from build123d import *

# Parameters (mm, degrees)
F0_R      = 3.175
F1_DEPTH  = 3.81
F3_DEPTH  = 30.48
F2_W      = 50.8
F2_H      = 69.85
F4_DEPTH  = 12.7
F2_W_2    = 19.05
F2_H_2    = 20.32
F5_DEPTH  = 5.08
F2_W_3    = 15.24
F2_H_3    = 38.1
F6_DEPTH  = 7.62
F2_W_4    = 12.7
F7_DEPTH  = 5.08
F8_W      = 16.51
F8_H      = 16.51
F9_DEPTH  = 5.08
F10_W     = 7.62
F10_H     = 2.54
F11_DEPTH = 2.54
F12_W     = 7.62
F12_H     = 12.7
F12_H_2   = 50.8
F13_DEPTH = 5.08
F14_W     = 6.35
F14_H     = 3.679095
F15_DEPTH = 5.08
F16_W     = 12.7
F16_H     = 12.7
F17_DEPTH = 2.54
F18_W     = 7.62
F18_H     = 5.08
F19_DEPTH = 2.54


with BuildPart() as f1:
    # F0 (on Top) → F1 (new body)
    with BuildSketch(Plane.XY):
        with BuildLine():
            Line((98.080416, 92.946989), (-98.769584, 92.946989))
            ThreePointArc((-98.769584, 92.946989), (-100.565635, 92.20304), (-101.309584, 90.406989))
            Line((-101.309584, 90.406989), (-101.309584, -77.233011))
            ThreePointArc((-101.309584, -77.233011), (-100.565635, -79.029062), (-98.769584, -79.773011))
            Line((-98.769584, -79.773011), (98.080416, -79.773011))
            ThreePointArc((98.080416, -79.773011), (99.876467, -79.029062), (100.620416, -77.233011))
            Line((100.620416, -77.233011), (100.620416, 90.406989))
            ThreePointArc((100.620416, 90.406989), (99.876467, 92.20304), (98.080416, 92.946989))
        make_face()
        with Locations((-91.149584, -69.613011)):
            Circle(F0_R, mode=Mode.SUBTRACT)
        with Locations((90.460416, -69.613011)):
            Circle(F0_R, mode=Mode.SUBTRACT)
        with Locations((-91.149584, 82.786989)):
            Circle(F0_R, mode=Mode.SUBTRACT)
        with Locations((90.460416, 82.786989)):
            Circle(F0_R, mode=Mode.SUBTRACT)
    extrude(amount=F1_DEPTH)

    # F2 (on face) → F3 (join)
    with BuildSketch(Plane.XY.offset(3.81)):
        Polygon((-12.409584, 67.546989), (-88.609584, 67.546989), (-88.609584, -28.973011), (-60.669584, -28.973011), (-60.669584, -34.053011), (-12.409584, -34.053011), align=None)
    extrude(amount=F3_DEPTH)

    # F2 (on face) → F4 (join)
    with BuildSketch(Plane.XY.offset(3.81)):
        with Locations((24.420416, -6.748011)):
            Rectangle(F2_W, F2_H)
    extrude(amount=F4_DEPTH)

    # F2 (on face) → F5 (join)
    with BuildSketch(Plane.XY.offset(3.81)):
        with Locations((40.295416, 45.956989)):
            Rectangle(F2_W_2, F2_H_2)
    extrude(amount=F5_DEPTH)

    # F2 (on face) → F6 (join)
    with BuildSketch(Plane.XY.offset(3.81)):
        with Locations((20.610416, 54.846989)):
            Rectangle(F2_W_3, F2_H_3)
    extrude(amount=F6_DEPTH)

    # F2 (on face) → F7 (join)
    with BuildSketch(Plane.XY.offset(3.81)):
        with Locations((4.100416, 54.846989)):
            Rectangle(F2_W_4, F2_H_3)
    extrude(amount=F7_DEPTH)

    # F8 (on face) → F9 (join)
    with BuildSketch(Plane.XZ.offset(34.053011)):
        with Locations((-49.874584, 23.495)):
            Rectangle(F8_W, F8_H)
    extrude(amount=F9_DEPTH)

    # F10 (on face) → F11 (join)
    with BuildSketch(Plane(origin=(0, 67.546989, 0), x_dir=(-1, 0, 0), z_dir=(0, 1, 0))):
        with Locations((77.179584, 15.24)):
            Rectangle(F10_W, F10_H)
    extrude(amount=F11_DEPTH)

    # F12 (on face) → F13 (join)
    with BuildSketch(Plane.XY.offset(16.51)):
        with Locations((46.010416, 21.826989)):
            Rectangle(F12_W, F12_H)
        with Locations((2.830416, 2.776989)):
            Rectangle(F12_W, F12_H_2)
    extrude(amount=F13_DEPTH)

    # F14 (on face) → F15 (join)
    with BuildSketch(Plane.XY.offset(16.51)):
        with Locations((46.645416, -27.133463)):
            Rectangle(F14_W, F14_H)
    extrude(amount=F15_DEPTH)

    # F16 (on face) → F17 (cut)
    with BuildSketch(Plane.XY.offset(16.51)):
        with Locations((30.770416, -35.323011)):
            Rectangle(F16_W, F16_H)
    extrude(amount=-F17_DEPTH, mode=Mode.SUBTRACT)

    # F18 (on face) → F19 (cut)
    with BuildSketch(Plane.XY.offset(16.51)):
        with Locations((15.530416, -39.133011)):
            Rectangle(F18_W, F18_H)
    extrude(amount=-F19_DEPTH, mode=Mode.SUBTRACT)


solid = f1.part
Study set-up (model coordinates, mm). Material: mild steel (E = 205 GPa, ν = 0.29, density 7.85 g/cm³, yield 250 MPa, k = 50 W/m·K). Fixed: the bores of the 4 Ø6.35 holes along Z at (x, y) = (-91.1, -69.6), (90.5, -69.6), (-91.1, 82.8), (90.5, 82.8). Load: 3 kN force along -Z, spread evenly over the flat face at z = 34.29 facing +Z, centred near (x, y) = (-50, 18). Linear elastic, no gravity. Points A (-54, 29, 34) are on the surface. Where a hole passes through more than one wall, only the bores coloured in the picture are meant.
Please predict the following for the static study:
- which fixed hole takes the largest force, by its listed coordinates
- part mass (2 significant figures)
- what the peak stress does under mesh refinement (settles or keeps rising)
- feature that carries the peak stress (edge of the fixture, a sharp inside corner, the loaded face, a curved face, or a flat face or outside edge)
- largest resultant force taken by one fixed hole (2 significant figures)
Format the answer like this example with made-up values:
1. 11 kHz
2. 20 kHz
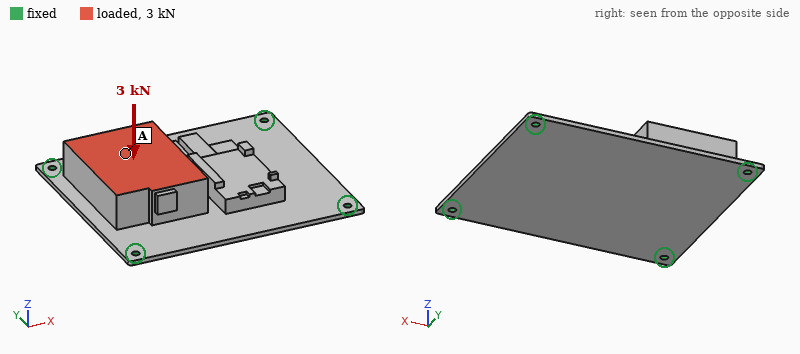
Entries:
1. (-91.1, 82.8)
2. 3.3 kg
3. keeps rising
4. edge of the fixture
5. 1.8 kN
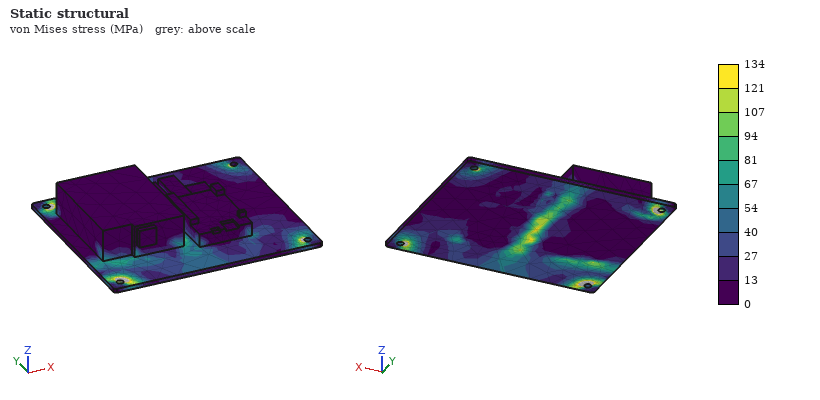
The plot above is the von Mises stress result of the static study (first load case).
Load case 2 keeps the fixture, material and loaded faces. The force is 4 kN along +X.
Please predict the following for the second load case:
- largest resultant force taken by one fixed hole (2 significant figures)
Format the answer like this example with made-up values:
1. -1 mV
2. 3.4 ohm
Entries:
1. 1.4 kN
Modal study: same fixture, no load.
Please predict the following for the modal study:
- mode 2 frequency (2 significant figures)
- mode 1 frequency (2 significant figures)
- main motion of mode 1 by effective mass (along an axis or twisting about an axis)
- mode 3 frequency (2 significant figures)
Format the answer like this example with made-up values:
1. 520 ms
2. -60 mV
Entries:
1. 680 Hz
2. 320 Hz
3. along Z
4. 1000 Hz
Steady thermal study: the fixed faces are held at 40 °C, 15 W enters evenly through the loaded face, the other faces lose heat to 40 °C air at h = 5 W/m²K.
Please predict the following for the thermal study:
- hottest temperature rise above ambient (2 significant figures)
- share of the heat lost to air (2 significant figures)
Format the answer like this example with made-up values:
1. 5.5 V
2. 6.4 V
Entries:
1. 18 K
2. 31 %
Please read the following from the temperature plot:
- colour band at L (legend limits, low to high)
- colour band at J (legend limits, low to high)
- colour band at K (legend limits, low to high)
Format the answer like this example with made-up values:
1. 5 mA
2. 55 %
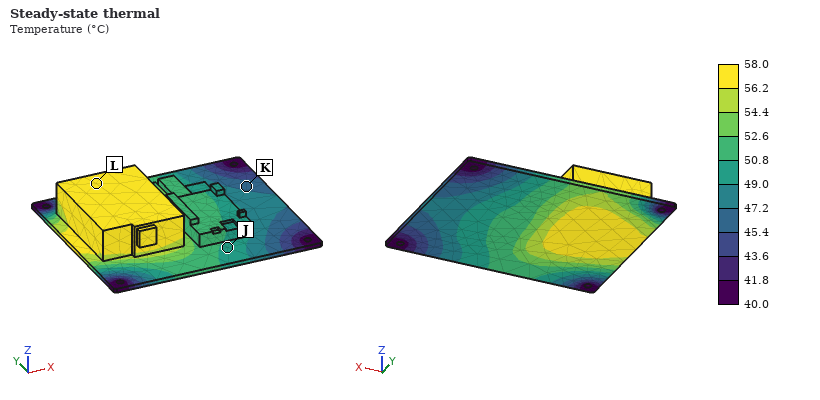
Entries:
1. 56.2 to 58.0 °C
2. 49.0 to 50.8 °C
3. 45.4 to 47.2 °C
